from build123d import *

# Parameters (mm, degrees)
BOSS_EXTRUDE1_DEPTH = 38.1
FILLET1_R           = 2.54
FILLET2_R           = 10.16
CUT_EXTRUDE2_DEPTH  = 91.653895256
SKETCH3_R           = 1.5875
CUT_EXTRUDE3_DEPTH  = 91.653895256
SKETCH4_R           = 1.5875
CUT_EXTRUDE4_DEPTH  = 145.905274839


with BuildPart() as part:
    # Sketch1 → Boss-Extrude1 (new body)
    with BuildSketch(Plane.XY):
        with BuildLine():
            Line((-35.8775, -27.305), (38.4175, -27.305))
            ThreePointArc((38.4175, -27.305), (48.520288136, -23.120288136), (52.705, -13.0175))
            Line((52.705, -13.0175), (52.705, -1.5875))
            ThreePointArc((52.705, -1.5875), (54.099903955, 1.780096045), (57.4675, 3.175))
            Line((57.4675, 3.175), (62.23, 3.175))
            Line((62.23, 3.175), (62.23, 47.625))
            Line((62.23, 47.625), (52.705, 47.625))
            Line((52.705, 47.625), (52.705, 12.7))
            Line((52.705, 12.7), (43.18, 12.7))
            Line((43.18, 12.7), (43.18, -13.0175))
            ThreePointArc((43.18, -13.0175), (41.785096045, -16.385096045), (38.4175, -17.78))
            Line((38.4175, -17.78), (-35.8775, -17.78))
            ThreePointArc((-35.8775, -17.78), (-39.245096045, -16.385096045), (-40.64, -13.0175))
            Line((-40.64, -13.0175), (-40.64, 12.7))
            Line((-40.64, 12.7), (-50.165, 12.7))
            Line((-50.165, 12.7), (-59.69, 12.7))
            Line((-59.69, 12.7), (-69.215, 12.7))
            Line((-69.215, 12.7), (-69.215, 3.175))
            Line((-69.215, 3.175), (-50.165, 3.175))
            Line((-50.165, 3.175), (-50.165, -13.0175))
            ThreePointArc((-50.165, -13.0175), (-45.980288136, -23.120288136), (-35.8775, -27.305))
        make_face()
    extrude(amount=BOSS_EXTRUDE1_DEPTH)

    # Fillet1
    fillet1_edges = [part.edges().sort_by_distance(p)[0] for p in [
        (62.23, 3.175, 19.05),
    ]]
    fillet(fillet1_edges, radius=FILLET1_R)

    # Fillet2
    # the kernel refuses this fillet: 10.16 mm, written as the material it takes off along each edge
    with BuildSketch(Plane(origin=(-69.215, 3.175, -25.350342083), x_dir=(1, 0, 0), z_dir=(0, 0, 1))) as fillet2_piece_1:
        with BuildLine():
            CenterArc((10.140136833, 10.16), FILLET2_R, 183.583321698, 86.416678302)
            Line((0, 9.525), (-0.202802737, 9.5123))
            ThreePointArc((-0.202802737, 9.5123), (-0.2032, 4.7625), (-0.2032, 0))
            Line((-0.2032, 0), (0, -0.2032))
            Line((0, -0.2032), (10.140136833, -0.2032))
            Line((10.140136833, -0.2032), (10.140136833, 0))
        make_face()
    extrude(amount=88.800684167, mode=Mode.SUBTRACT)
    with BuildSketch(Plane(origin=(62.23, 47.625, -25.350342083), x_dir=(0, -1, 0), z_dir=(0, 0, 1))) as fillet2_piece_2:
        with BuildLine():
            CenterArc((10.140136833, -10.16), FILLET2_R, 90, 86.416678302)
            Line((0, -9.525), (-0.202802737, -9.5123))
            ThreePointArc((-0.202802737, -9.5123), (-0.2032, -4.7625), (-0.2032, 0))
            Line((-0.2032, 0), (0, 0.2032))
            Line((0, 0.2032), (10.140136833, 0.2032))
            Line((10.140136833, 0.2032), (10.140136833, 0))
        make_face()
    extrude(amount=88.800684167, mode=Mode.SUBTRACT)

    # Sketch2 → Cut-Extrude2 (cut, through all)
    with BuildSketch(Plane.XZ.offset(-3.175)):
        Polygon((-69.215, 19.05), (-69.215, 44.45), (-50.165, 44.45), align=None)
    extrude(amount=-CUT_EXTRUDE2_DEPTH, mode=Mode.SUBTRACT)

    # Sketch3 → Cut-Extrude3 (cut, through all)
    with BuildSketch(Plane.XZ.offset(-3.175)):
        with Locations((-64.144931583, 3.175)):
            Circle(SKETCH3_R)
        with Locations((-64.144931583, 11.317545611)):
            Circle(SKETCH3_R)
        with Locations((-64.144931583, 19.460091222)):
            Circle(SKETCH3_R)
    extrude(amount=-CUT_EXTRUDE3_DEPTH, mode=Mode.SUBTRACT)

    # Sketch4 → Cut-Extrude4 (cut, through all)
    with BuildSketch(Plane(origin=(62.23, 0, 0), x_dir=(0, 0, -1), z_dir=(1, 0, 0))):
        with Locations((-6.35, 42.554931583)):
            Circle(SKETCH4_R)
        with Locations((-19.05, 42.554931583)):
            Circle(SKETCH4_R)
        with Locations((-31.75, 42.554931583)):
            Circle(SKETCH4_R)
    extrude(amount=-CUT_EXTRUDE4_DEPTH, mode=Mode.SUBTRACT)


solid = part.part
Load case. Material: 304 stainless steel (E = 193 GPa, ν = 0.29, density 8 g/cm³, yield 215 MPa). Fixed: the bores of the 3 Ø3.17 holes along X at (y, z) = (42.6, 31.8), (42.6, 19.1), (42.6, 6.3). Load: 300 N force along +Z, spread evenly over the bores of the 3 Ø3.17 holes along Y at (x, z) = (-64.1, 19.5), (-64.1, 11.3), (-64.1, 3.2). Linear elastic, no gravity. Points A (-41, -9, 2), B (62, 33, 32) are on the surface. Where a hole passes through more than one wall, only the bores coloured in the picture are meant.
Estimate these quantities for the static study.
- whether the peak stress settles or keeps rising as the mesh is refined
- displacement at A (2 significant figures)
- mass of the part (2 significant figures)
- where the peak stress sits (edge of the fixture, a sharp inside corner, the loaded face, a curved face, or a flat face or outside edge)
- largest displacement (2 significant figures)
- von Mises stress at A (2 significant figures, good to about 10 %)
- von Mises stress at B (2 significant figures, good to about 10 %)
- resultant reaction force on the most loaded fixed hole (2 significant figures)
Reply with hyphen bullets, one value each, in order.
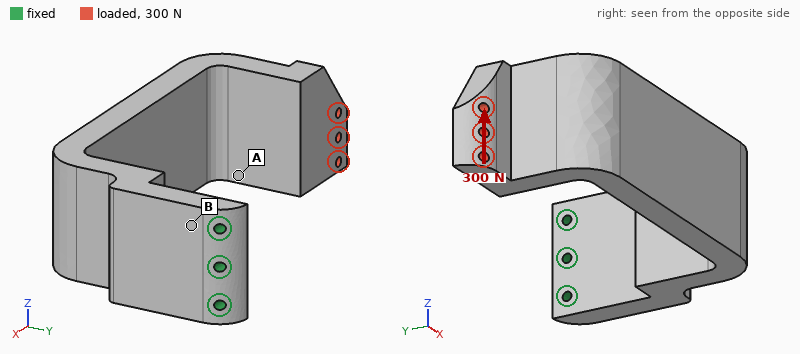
- keeps rising
- 0.25 mm
- 610 g
- edge of the fixture
- 0.36 mm
- 6.1 MPa
- 43 MPa
- 1.2 kN
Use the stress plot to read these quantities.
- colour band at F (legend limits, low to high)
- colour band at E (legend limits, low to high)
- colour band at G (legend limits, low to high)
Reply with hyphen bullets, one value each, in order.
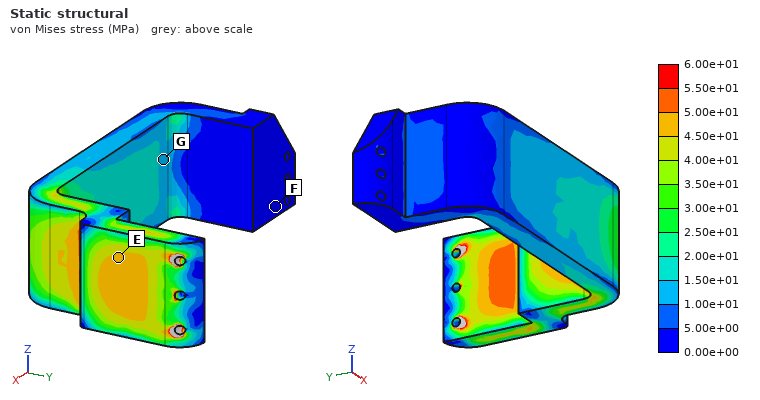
- 0.00e+00 to 5.00e+00 MPa
- 4.50e+01 to 5.00e+01 MPa
- 1.00e+01 to 1.50e+01 MPa
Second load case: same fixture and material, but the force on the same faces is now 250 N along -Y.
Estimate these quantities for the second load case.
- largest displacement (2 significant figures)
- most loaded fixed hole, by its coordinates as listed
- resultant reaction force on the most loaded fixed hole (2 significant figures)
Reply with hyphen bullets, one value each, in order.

- 0.67 mm
- (42.6, 19.1)
- 230 N
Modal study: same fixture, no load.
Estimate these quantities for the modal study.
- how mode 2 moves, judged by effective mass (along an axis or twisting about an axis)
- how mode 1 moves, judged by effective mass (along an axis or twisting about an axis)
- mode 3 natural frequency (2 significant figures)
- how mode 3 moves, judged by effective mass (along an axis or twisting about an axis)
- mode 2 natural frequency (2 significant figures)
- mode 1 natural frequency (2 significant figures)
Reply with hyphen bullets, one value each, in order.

- along Z
- along Y
- 760 Hz
- along X
- 390 Hz
- 250 Hz
